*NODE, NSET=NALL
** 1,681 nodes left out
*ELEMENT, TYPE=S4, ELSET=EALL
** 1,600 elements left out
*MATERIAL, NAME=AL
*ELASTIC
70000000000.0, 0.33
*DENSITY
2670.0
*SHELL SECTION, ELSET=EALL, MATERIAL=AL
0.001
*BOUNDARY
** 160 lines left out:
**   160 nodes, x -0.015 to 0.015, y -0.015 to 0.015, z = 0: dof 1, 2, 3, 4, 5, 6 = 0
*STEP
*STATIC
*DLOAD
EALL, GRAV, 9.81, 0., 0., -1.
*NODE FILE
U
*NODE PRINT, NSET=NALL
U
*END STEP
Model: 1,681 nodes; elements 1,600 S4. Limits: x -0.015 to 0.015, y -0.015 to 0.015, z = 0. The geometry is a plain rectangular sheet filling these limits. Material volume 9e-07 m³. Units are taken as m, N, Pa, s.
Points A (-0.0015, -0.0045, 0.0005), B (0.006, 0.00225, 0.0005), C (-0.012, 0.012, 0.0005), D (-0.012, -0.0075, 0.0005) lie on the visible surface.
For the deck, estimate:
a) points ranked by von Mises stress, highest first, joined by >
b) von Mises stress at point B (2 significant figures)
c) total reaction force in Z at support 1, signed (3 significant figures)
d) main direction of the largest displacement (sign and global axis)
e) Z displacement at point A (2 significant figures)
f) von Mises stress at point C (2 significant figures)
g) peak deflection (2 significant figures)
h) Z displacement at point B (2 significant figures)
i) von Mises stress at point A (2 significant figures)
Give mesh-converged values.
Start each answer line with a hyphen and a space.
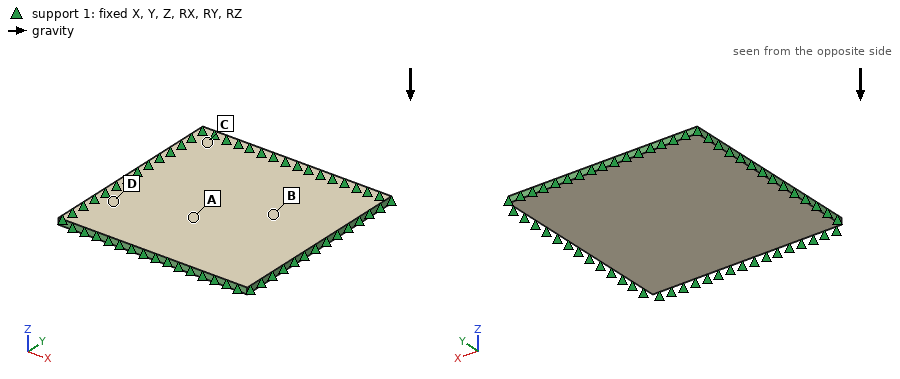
- A > B > D > C
- 2300 Pa
- 0.0236 N
- -Z
- -3.4e-09 m
- 1500 Pa
- 4.1e-09 m
- -2.9e-09 m
- 2700 Pa
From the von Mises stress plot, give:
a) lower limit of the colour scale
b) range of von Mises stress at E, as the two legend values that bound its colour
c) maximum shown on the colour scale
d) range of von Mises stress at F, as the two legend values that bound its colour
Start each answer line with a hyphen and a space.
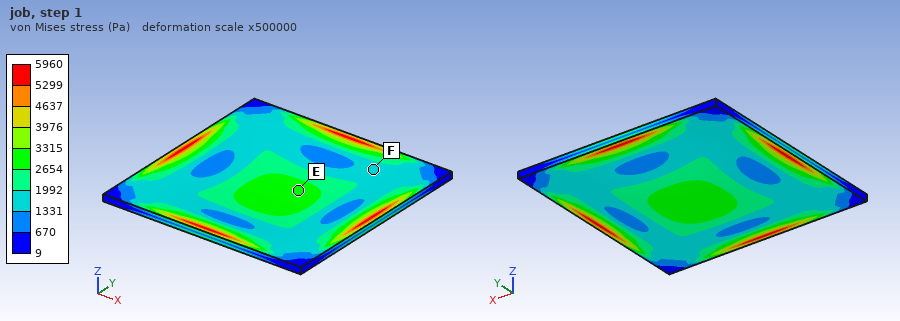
- 9 Pa
- 2654 to 3315 Pa
- 5960 Pa
- 1331 to 1992 Pa
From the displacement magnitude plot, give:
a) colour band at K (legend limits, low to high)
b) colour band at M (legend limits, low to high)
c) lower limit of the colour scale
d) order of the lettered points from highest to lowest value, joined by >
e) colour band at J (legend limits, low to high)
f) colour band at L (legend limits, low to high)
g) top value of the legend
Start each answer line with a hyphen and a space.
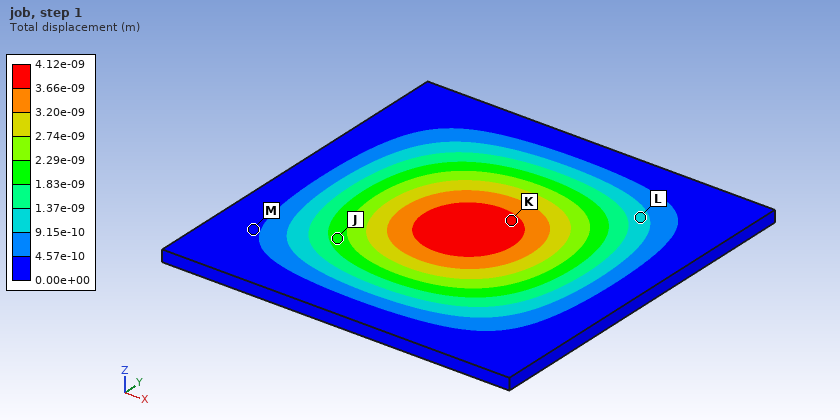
- 3.66e-09 to 4.12e-09 m
- 0.00e+00 to 4.57e-10 m
- 0.00e+00 m
- K > J > L > M
- 1.83e-09 to 2.29e-09 m
- 9.15e-10 to 1.37e-09 m
- 4.12e-09 m
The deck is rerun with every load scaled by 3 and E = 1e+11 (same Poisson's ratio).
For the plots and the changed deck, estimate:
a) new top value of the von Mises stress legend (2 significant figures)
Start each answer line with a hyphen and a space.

- 18000 Pa
